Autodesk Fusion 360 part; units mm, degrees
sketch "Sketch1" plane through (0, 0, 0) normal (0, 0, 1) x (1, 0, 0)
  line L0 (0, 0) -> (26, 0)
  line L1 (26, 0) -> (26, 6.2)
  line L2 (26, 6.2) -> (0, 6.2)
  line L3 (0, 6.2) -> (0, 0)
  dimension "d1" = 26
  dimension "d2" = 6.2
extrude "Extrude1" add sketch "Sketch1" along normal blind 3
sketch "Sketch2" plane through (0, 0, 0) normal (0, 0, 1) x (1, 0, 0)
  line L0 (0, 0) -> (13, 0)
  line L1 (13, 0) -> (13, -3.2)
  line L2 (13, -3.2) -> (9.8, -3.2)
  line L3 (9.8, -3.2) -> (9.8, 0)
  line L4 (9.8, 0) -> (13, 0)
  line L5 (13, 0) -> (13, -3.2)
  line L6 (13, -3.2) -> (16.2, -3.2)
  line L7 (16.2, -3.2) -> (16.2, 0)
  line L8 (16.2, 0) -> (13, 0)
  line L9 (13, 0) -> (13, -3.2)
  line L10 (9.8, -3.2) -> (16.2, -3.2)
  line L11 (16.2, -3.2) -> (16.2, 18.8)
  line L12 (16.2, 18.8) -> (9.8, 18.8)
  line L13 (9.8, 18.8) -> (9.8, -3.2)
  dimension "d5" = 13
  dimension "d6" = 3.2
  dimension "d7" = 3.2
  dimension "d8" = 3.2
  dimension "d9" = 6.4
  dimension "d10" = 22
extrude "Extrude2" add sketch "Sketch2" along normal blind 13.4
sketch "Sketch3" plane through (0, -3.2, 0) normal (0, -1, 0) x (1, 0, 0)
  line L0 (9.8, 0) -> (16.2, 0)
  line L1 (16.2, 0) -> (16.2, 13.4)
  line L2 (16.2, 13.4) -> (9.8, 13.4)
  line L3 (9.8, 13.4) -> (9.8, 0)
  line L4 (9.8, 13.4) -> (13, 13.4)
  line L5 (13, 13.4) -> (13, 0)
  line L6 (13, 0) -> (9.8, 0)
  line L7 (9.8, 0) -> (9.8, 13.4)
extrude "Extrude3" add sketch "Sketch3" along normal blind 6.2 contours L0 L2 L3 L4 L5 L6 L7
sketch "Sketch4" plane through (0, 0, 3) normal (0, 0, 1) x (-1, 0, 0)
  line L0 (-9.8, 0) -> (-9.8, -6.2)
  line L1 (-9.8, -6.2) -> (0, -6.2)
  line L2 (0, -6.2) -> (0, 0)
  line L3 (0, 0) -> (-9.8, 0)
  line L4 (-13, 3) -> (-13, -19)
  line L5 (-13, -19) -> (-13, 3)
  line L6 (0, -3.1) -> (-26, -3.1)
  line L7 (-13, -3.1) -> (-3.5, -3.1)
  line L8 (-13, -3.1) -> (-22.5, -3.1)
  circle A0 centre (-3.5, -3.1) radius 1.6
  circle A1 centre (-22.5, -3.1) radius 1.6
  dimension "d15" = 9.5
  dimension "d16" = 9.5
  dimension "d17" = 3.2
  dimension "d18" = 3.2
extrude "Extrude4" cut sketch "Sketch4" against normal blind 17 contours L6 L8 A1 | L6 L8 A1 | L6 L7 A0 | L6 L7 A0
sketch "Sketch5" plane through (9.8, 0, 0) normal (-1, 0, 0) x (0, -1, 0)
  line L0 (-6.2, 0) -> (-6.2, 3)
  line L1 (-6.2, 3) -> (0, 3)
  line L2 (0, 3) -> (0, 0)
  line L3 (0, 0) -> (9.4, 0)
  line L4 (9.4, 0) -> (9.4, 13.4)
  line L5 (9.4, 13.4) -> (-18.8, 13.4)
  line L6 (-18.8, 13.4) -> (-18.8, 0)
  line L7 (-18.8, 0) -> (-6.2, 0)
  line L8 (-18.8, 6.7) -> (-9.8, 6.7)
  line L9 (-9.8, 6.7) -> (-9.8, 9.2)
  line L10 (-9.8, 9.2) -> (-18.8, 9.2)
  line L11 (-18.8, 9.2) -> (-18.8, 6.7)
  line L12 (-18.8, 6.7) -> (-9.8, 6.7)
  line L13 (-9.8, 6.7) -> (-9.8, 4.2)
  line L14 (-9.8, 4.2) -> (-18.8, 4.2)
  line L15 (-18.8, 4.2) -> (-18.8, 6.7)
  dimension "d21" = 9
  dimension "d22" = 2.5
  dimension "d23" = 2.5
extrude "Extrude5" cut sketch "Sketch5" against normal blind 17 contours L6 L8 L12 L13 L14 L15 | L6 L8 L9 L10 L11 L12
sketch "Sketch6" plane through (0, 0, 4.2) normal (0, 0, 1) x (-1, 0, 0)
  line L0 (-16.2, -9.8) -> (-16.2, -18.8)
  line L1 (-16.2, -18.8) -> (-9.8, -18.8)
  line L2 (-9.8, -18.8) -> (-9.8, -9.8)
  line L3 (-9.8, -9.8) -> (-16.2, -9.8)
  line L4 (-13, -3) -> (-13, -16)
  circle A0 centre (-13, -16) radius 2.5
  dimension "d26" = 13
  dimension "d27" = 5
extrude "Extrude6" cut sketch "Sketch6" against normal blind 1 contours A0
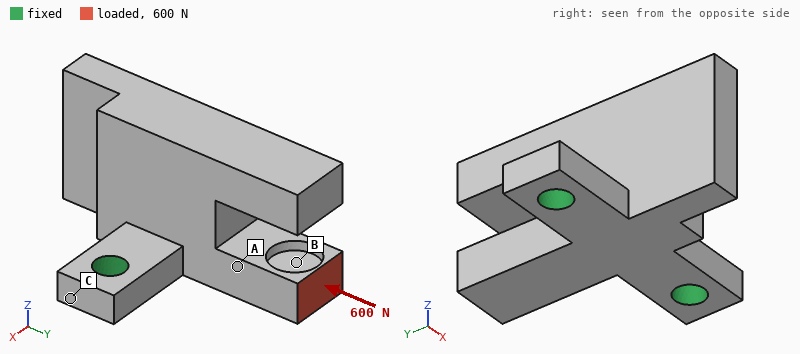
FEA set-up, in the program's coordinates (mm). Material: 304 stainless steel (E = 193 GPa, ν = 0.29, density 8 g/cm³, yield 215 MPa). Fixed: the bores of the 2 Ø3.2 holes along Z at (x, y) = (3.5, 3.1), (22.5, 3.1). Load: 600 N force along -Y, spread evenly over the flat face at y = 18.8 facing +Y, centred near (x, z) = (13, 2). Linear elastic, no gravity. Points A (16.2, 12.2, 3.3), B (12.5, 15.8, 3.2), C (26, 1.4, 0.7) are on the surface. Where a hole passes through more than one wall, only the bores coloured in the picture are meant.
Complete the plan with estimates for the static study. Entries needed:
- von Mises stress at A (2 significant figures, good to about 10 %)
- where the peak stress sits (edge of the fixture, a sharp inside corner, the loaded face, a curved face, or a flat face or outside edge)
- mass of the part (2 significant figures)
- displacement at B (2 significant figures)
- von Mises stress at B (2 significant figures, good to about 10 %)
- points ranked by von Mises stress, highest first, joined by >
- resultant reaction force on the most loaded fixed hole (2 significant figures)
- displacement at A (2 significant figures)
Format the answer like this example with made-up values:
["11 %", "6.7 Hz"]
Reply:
["28 MPa", "the loaded face", "17 g", "6.0 µm", "44 MPa", "B > A > C", "300 N", "4.7 µm"]
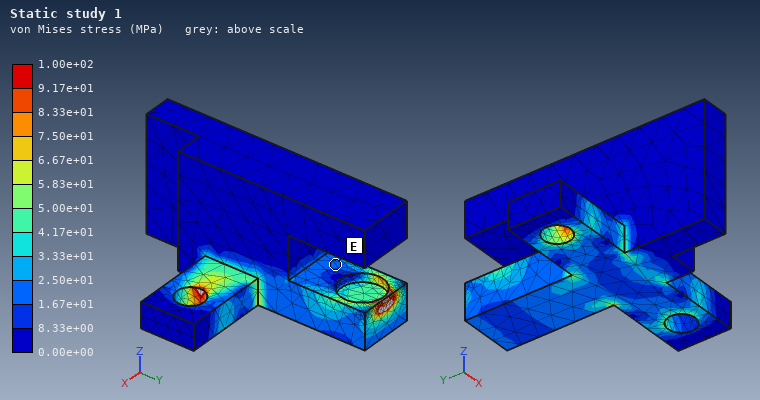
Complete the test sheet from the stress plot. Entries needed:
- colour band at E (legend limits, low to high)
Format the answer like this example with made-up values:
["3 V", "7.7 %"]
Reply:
["1.67e+01 to 2.50e+01 MPa"]
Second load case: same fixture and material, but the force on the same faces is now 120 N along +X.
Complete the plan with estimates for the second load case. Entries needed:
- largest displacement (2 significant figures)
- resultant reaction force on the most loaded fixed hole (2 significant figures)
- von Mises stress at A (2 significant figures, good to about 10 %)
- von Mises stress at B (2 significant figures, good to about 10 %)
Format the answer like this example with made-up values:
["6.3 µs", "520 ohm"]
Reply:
["9.4 µm", "140 N", "28 MPa", "23 MPa"]
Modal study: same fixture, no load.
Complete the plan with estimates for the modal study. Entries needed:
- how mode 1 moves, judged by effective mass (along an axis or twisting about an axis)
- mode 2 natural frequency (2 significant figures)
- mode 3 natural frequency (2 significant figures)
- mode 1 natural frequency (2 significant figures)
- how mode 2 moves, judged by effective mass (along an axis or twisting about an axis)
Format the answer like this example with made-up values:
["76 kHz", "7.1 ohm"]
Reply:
["along Y", "11 kHz", "15 kHz", "4300 Hz", "along X"]
